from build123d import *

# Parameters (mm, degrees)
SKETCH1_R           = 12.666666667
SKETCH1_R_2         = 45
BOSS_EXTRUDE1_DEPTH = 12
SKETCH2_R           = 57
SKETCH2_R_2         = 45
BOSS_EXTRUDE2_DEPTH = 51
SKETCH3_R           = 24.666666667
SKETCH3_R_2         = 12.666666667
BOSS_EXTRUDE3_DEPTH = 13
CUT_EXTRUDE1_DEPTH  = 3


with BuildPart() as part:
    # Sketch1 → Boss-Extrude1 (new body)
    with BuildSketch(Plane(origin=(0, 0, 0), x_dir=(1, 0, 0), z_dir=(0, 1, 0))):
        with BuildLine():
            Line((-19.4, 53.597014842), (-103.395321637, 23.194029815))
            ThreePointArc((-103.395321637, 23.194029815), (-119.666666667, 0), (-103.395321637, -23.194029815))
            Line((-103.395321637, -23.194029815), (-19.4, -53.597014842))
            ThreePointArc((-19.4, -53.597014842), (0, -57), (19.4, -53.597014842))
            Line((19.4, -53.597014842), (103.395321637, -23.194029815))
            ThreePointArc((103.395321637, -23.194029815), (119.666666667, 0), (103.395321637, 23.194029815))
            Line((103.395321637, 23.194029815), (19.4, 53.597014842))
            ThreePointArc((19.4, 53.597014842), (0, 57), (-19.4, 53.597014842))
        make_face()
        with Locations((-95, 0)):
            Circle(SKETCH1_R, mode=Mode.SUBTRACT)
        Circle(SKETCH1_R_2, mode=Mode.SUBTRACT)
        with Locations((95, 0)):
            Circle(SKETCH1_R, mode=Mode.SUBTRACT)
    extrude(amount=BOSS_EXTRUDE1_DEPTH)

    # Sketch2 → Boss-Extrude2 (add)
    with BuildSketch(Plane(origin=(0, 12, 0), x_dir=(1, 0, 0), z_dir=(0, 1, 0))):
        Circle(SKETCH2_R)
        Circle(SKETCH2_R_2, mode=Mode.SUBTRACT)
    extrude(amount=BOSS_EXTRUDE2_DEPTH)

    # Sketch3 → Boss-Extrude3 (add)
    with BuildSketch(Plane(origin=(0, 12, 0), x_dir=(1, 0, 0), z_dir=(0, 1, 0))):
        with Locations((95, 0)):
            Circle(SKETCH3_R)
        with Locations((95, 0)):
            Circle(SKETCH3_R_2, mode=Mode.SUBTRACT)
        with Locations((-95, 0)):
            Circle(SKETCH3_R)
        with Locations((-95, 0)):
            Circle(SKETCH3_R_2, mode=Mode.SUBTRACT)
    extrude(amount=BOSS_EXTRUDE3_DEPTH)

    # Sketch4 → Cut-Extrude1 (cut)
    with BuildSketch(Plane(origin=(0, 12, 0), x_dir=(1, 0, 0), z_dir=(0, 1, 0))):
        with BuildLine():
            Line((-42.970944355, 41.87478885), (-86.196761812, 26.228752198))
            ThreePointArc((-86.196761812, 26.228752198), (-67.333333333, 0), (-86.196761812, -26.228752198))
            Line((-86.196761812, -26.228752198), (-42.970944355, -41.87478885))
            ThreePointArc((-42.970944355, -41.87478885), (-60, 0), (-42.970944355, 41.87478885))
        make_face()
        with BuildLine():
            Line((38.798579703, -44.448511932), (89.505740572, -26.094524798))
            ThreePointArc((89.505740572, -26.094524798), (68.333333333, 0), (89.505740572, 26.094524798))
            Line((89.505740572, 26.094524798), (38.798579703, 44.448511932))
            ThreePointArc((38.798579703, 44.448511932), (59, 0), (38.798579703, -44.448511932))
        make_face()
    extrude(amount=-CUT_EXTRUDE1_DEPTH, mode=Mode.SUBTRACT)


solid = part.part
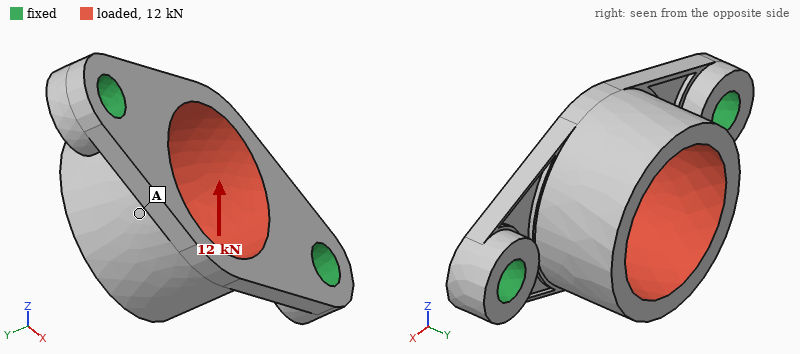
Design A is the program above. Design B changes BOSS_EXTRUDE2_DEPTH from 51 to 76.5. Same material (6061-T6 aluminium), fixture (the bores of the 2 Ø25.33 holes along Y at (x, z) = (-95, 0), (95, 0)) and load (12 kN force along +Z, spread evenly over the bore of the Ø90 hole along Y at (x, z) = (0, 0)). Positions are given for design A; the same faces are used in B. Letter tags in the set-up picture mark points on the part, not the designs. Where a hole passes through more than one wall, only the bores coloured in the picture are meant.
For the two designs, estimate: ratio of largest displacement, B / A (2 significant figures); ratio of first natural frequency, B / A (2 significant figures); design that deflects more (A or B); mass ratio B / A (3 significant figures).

1.8
0.70
B
1.28
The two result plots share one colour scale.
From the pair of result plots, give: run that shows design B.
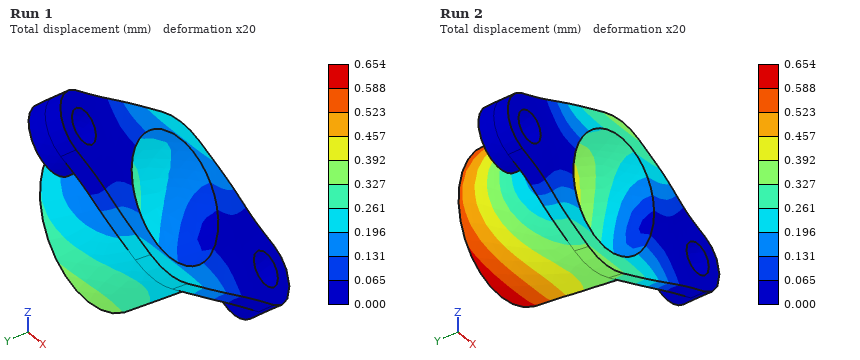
Run 2
